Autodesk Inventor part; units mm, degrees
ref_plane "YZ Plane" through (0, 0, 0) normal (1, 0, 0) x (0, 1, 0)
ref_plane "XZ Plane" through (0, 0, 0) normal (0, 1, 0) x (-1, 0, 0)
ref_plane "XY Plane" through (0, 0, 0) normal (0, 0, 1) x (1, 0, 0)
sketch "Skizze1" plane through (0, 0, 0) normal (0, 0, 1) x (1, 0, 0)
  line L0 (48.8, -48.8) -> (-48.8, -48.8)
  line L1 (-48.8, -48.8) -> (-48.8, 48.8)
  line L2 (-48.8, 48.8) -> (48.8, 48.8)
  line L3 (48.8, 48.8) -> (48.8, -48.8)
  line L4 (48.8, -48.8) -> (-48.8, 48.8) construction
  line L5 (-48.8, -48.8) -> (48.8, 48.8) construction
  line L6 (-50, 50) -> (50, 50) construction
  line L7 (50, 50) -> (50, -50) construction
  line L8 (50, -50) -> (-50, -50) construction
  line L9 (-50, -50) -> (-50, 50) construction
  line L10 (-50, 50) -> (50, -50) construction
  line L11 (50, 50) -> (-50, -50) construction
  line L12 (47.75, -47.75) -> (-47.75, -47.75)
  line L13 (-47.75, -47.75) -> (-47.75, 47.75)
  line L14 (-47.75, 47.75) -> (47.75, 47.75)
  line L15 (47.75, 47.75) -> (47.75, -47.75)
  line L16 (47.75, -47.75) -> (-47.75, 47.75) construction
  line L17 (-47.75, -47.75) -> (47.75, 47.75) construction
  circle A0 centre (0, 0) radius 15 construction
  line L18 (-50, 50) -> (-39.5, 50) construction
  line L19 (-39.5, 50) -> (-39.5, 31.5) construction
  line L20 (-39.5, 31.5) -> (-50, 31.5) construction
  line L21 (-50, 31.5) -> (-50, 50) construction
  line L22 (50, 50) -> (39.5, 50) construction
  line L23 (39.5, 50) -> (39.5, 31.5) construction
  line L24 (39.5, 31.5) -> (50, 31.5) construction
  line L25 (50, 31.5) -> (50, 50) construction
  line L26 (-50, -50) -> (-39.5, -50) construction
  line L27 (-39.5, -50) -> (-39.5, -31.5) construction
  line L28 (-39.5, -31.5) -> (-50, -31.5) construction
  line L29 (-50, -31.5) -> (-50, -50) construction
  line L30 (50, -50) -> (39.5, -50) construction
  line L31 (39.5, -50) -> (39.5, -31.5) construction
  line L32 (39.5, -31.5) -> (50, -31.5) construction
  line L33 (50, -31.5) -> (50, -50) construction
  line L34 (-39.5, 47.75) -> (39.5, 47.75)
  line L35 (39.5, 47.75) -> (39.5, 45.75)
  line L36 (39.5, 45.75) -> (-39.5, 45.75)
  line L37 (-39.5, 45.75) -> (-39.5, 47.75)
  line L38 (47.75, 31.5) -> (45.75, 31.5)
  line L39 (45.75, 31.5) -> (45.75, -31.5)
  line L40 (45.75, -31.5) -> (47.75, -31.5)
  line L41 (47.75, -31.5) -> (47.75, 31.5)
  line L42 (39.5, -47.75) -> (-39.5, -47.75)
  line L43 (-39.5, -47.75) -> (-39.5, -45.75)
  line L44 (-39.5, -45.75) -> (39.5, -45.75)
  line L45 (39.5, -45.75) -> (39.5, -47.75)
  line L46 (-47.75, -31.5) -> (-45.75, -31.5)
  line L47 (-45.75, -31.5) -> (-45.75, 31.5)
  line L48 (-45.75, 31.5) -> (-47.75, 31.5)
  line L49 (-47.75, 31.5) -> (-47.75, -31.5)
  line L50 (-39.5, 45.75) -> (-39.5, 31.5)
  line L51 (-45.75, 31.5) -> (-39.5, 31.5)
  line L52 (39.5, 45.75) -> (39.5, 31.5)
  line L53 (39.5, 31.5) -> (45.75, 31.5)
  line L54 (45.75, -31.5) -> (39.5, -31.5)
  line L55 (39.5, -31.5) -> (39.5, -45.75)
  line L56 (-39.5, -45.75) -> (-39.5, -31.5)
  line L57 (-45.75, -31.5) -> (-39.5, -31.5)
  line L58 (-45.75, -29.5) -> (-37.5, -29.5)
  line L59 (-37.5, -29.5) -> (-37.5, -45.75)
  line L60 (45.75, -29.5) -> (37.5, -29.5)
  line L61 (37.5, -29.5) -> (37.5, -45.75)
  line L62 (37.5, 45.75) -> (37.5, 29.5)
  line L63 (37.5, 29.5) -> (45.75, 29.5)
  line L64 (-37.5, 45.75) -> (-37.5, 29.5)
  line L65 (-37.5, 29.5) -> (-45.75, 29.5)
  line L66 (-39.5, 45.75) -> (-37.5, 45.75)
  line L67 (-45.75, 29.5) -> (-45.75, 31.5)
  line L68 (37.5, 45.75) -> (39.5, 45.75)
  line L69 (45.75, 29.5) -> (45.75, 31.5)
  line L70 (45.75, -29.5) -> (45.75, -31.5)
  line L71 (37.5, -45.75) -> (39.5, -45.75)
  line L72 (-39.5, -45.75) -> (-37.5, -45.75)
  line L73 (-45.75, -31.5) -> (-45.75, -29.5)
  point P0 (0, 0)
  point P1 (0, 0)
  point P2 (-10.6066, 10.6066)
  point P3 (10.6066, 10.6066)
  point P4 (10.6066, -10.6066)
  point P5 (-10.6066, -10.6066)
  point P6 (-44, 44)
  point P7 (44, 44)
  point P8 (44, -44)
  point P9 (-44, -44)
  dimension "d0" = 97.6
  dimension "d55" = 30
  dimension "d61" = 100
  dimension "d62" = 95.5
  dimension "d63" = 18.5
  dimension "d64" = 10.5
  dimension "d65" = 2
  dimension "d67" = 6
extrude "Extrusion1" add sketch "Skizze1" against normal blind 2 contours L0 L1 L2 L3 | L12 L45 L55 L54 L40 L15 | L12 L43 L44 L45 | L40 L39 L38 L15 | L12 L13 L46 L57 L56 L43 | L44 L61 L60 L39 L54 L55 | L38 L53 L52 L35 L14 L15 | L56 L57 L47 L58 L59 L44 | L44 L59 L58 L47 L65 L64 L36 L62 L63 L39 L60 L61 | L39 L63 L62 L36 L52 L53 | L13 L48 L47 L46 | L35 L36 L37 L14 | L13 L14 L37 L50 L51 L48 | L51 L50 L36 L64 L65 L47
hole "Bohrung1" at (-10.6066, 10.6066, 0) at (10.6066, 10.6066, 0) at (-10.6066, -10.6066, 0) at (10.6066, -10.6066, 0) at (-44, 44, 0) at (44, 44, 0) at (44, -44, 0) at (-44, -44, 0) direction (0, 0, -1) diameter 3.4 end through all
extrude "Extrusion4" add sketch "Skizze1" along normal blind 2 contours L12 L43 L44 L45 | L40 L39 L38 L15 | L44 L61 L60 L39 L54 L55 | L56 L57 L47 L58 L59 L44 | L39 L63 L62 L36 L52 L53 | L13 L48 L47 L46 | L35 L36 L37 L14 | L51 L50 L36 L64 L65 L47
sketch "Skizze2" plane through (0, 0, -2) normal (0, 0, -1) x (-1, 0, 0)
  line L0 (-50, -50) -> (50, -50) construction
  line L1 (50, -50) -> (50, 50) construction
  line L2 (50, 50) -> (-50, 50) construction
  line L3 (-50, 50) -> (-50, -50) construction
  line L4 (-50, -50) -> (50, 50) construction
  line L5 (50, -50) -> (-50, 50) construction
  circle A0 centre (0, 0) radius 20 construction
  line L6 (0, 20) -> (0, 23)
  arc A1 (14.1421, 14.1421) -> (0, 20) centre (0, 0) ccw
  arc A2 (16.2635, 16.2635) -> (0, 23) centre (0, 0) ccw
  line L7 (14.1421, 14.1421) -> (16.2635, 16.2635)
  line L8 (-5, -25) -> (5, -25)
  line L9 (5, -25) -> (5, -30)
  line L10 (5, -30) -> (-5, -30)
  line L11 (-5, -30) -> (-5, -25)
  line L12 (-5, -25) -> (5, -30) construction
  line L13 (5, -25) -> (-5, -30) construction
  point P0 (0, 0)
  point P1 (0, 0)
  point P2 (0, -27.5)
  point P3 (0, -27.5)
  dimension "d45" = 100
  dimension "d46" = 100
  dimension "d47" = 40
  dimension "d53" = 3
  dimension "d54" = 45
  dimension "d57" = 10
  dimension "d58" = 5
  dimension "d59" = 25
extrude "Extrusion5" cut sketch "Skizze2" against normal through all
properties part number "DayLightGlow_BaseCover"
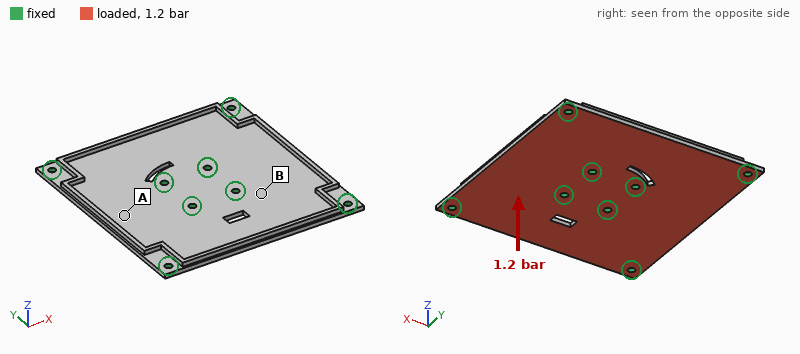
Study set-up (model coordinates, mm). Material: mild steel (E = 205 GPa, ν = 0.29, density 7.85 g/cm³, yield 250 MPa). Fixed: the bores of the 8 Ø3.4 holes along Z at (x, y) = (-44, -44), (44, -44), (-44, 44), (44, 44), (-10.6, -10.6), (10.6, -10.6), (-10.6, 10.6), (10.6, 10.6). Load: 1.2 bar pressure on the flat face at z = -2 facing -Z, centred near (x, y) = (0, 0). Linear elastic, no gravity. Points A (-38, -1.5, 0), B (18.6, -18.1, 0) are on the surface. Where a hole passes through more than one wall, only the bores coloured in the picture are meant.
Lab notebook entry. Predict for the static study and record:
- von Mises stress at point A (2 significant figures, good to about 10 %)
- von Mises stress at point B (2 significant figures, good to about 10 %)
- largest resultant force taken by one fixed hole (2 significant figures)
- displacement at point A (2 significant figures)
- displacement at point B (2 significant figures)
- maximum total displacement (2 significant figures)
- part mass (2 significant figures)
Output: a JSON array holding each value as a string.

["11 MPa", "26 MPa", "160 N", "33 µm", "10 µm", "48 µm", "160 g"]
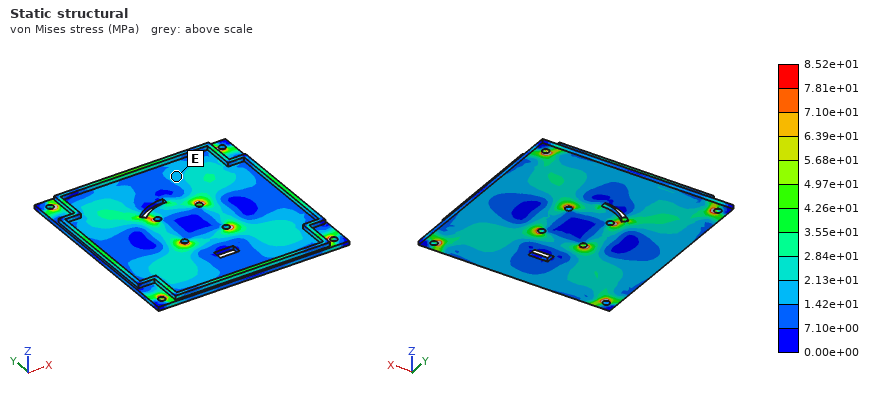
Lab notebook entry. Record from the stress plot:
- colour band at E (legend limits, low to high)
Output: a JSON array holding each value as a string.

["1.42e+01 to 2.13e+01 MPa"]
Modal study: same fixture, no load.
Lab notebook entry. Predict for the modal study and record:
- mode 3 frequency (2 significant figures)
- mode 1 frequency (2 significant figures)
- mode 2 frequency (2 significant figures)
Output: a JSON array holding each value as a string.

["2400 Hz", "2100 Hz", "2300 Hz"]
